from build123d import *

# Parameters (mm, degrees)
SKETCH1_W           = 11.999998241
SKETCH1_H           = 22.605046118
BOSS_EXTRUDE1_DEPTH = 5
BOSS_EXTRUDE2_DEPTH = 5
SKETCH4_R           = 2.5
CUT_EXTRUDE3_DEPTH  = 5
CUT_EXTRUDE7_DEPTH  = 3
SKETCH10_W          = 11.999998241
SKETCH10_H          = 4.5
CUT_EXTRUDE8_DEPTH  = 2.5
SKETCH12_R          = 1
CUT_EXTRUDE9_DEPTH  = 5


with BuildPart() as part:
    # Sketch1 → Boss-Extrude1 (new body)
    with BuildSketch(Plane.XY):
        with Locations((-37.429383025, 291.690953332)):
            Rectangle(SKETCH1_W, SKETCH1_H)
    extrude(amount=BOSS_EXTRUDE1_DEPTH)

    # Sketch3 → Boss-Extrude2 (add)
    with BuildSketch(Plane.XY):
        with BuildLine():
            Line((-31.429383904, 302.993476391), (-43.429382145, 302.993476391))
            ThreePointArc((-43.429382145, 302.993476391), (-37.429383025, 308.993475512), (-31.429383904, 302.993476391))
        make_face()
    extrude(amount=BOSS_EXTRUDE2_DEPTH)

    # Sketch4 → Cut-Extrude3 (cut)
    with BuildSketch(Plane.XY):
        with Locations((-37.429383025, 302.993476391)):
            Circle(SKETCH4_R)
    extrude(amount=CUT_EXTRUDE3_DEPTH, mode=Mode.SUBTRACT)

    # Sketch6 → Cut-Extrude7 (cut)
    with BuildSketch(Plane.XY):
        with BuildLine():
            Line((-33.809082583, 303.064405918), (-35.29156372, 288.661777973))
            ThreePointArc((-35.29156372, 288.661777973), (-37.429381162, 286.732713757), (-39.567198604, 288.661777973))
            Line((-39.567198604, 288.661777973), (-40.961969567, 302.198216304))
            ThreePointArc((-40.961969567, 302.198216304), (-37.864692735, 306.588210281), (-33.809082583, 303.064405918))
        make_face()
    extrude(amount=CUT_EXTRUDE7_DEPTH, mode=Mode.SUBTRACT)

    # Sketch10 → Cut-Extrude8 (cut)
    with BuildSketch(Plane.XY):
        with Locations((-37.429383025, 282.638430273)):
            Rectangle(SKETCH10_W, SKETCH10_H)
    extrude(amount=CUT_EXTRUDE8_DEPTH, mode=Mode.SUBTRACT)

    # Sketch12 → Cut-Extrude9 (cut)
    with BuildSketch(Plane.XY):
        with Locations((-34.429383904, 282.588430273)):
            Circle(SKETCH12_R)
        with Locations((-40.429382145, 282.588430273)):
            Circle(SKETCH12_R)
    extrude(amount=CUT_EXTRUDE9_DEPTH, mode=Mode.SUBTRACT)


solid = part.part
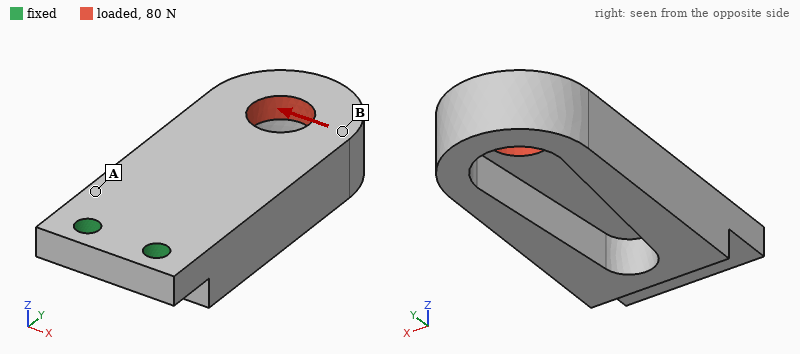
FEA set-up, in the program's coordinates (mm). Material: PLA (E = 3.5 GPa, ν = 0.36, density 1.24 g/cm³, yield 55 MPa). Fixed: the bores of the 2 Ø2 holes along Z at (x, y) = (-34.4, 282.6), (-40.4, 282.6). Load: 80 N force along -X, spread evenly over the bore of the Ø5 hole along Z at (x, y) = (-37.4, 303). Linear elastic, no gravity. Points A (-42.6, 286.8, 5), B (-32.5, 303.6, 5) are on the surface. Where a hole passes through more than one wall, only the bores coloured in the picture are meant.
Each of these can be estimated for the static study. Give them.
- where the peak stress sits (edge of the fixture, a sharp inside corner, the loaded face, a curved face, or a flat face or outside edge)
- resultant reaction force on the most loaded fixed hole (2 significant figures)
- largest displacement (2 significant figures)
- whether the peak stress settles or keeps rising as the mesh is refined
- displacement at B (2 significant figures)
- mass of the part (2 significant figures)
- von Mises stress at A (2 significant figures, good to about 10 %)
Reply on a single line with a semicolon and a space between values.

edge of the fixture; 220 N; 0.31 mm; keeps rising; 0.26 mm; 1.4 g; 17 MPa
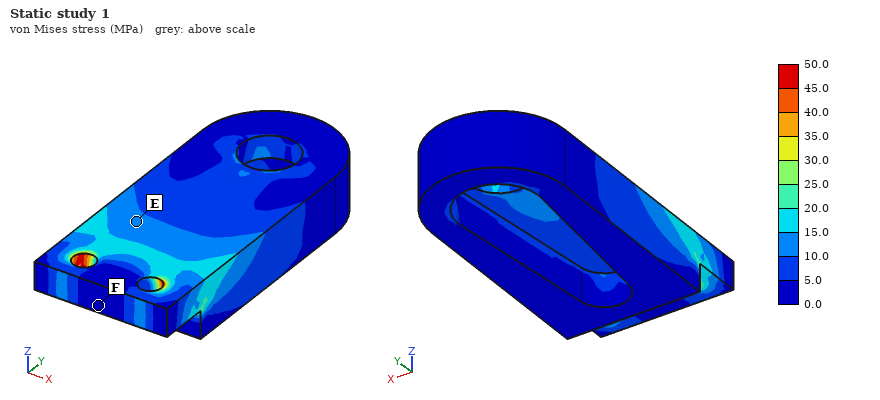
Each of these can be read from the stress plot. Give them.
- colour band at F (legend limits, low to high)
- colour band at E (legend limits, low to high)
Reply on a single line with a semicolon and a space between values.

0.0 to 5.0 MPa; 10.0 to 15.0 MPa
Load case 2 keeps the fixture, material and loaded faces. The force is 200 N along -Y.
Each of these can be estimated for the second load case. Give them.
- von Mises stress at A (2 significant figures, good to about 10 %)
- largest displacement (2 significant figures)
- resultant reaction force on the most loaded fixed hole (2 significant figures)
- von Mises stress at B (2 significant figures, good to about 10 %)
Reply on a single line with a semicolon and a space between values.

9.6 MPa; 0.26 mm; 100 N; 5.1 MPa
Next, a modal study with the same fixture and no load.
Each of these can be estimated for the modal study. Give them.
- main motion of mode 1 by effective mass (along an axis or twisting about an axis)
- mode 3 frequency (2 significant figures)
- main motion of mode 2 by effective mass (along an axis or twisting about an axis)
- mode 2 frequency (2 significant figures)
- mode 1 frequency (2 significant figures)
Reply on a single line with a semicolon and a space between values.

along Z; 4700 Hz; along X; 3600 Hz; 1300 Hz
